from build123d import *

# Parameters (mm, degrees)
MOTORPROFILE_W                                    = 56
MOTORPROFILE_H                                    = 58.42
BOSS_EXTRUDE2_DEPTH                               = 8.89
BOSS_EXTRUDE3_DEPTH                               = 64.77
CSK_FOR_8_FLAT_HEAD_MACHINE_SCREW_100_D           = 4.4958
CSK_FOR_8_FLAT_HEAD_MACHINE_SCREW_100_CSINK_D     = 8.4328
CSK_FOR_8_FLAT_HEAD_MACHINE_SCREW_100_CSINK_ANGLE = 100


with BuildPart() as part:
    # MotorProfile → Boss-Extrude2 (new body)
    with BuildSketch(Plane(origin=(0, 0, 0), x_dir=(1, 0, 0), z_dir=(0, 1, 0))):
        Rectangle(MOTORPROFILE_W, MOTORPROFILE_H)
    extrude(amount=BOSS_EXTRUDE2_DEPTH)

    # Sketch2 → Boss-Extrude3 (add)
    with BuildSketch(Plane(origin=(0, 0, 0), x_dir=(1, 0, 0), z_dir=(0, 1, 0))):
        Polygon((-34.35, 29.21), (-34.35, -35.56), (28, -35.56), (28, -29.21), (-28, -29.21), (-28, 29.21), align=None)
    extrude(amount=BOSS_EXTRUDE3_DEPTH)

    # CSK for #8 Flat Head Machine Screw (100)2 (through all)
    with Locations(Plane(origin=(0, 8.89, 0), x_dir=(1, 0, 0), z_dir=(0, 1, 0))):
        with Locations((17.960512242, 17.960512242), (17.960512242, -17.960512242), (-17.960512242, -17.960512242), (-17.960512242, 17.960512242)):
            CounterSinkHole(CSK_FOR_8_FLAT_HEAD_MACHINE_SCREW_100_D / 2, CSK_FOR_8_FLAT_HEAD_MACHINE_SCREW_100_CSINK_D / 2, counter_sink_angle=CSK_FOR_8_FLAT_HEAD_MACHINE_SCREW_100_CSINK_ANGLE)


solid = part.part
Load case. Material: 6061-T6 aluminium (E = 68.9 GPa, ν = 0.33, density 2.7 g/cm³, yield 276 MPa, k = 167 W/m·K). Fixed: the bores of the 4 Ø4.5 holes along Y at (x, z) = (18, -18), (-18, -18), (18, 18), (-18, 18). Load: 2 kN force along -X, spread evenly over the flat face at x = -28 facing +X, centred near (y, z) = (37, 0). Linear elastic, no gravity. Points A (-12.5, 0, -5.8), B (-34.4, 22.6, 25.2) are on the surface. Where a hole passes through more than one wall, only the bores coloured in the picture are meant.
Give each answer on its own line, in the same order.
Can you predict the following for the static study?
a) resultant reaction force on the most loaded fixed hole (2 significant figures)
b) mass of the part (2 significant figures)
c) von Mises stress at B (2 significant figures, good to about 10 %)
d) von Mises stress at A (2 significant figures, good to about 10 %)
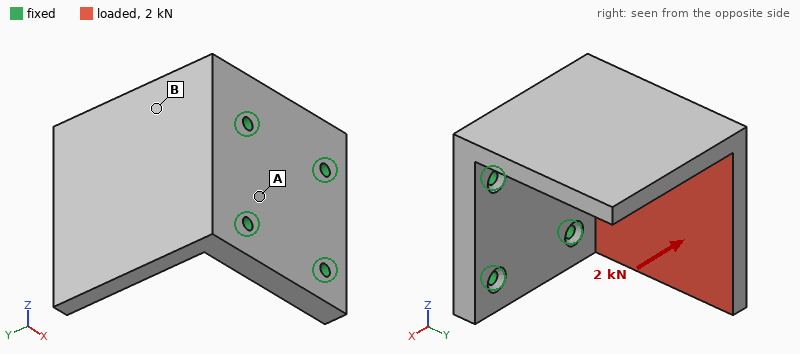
1.5 kN
210 g
26 MPa
11 MPa
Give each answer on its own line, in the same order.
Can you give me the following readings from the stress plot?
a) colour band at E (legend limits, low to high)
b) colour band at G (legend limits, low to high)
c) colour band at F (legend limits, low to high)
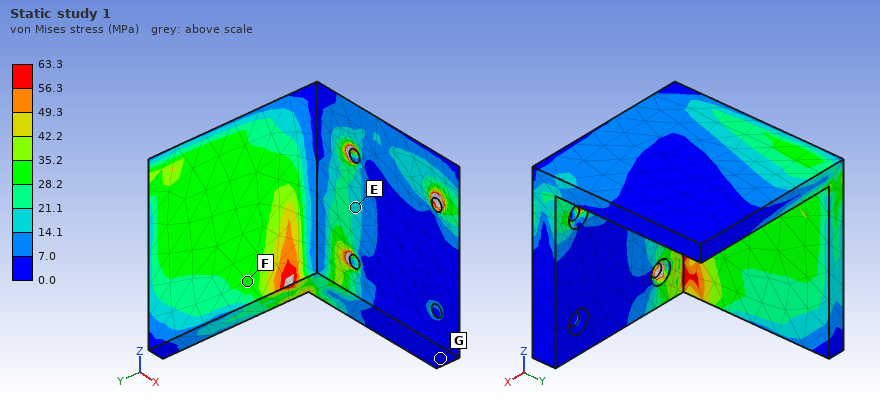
14.1 to 21.1 MPa
0.0 to 7.0 MPa
28.2 to 35.2 MPa
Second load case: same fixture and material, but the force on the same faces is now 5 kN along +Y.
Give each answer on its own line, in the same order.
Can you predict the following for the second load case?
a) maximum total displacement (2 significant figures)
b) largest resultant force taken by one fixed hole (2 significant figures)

52 µm
2.8 kN
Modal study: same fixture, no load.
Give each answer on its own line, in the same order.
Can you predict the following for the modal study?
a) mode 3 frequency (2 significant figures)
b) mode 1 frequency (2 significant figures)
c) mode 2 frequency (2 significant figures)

3500 Hz
1900 Hz
2600 Hz
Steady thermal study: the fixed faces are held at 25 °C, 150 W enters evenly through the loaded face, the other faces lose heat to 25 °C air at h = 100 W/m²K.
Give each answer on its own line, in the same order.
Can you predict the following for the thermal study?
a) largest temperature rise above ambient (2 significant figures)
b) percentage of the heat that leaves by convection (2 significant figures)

62 K
25 %
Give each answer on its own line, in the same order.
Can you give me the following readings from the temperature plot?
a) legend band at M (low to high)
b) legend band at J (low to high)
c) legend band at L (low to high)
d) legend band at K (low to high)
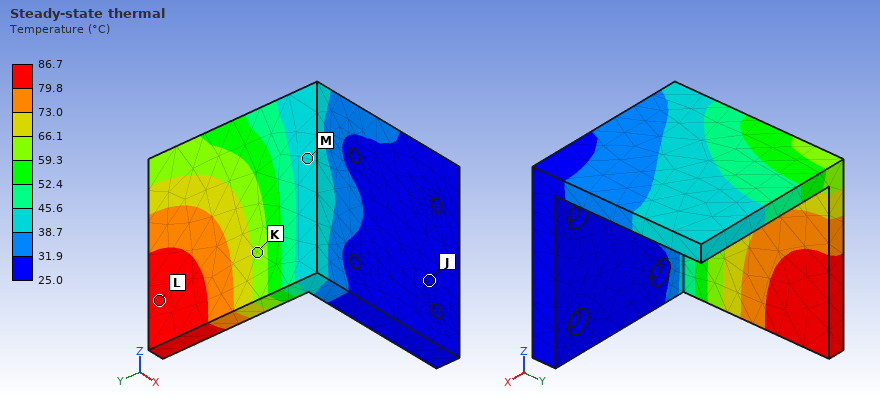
38.7 to 45.6 °C
25.0 to 31.9 °C
79.8 to 86.7 °C
59.3 to 66.1 °C
